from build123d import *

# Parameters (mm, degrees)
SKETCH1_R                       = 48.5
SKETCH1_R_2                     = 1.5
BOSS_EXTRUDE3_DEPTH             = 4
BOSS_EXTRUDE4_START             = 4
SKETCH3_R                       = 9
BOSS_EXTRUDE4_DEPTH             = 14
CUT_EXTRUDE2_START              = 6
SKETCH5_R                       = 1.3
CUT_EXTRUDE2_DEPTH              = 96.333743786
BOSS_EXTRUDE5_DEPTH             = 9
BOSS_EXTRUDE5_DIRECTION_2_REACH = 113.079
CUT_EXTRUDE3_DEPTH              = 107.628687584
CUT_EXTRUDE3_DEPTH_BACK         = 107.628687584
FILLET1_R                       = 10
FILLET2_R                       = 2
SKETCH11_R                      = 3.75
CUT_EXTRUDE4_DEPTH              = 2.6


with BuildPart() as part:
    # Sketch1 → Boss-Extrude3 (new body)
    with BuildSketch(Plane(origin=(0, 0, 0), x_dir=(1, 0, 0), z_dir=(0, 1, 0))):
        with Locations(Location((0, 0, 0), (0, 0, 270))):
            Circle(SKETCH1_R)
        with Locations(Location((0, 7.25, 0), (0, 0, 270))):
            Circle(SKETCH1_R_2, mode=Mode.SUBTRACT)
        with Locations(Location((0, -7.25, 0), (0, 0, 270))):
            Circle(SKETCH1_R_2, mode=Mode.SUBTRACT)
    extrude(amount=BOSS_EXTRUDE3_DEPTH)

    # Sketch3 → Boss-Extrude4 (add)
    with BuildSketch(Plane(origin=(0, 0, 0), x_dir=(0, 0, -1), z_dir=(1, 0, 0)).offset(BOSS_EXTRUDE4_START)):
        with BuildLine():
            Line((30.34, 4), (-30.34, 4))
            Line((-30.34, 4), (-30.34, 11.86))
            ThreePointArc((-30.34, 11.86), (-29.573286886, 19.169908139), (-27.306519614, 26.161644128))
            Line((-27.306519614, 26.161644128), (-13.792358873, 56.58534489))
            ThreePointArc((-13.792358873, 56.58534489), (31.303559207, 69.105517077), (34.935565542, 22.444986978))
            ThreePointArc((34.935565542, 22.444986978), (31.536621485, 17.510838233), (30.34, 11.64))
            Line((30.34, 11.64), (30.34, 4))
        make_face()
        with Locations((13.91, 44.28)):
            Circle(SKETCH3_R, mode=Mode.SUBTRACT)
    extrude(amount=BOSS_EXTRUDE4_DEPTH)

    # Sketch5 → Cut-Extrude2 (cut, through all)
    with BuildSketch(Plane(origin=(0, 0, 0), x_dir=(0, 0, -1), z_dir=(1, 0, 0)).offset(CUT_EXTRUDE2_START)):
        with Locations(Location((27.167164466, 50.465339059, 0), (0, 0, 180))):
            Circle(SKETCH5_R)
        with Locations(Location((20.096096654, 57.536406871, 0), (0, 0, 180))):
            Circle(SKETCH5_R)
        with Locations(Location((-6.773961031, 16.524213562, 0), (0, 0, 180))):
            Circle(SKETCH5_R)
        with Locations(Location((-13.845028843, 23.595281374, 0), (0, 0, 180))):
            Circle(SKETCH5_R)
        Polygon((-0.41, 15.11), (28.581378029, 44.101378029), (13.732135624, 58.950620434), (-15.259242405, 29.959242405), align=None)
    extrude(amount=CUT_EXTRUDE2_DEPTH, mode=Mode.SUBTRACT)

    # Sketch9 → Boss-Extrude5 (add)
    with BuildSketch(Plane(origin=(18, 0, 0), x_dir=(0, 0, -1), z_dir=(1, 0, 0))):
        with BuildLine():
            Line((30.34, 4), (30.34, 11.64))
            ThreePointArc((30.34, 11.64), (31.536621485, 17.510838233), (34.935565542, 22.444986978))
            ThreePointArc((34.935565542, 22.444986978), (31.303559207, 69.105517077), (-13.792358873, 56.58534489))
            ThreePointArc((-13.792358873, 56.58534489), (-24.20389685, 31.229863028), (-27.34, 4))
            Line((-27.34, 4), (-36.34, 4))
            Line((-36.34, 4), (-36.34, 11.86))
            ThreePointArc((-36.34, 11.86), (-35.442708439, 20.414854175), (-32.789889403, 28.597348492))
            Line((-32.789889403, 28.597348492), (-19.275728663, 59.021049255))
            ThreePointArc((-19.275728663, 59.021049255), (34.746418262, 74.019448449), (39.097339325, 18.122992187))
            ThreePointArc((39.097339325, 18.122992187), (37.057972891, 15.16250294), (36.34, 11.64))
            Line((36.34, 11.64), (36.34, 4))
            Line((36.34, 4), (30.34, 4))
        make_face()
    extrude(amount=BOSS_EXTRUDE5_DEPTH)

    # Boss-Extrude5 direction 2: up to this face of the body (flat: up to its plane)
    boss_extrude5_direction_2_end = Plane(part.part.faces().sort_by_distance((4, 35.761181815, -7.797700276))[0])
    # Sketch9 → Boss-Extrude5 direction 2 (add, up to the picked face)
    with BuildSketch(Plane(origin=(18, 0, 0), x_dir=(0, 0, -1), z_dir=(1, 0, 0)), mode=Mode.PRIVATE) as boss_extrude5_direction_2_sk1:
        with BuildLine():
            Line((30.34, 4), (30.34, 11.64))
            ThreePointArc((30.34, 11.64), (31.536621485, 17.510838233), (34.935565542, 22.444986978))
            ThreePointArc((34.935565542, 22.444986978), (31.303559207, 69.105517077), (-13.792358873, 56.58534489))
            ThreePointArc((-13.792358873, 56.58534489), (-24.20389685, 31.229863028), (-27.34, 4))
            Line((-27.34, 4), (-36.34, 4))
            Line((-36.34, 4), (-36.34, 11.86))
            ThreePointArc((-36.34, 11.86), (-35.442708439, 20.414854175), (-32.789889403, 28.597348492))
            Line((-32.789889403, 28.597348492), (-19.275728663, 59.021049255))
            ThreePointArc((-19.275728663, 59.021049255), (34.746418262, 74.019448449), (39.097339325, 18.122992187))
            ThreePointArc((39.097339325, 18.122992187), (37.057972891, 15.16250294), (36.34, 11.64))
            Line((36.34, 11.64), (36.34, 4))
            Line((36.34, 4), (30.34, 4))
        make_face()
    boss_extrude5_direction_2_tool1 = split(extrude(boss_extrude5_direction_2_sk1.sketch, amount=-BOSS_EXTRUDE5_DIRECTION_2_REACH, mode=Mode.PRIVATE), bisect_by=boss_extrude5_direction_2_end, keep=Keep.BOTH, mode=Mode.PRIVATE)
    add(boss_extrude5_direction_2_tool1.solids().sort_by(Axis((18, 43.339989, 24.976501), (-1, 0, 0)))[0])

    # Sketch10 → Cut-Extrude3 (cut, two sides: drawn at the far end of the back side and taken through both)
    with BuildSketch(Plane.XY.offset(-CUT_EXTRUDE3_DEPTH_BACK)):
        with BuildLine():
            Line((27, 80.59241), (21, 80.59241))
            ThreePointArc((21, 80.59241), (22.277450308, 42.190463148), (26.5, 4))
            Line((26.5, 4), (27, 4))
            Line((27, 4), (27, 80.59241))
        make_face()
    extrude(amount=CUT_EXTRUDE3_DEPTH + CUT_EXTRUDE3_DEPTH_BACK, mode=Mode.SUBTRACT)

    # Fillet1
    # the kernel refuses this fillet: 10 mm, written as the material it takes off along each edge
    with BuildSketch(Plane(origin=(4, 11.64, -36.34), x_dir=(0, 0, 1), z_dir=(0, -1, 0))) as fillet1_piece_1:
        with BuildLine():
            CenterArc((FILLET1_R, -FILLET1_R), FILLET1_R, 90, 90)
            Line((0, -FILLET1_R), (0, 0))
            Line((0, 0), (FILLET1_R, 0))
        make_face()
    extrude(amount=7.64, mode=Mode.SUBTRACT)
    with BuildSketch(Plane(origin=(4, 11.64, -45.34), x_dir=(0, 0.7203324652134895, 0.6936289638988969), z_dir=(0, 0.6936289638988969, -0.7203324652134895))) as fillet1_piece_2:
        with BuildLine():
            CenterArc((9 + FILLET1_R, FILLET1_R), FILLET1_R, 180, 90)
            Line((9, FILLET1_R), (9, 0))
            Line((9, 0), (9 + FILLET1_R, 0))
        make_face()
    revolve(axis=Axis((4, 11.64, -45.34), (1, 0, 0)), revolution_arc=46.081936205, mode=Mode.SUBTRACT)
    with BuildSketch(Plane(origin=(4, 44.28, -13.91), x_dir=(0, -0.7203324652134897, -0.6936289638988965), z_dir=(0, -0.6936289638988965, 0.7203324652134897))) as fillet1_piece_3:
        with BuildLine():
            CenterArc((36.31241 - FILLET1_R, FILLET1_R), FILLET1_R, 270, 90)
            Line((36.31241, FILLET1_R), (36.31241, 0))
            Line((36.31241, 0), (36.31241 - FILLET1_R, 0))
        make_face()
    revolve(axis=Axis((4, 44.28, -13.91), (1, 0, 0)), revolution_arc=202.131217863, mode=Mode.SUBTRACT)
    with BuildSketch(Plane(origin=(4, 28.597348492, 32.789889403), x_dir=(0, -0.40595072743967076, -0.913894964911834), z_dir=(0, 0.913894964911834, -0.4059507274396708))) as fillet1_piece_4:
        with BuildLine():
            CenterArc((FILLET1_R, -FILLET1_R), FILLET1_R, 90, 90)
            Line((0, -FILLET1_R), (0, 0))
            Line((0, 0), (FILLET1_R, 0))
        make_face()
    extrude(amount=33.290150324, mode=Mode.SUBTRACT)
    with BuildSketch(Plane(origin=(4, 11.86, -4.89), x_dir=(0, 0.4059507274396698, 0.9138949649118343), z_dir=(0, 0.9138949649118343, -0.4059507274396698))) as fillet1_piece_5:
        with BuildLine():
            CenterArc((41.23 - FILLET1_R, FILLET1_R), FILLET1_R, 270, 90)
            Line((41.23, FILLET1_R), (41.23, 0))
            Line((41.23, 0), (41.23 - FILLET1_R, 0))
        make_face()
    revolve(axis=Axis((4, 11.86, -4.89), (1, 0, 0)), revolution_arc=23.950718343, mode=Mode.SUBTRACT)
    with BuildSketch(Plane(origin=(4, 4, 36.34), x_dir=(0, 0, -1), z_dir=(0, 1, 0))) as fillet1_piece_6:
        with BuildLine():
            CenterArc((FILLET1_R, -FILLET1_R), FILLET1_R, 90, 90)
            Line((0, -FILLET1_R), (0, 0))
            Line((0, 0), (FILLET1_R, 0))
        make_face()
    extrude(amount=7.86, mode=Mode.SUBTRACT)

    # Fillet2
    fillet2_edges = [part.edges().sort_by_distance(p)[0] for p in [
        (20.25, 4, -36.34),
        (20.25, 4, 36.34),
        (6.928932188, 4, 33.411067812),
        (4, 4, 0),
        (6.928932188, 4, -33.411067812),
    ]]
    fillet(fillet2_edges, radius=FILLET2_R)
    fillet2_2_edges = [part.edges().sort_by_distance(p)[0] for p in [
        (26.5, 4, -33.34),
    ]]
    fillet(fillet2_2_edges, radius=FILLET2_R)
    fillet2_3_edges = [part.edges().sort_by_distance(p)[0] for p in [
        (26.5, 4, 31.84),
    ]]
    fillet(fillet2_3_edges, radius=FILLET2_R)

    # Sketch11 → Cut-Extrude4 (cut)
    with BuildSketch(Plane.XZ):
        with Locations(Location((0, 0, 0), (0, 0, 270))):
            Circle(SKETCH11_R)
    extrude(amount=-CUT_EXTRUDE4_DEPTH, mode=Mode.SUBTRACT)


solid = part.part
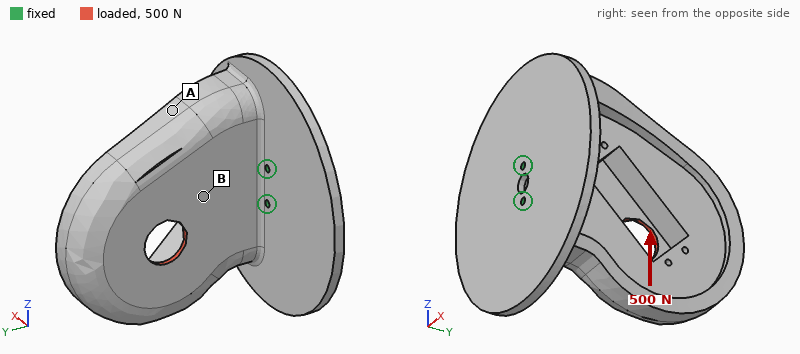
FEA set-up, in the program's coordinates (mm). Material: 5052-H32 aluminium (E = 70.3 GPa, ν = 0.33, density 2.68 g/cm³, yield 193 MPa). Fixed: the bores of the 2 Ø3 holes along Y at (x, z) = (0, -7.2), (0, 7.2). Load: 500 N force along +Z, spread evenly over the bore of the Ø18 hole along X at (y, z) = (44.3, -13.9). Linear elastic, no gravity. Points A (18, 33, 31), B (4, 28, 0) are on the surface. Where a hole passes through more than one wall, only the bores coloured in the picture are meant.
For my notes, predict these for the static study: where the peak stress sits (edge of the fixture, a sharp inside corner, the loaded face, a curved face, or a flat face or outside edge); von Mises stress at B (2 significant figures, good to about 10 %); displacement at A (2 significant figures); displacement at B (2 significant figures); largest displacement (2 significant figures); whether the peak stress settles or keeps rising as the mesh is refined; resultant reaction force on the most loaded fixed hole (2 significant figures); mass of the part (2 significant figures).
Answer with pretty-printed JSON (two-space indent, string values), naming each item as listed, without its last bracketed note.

{
  "where the peak stress sits": "edge of the fixture",
  "von Mises stress at B": "7.9 MPa",
  "displacement at A": "53 µm",
  "displacement at B": "34 µm",
  "largest displacement": "100 µm",
  "whether the peak stress settles or keeps rising as the mesh is refined": "keeps rising",
  "resultant reaction force on the most loaded fixed hole": "1.2 kN",
  "mass of the part": "250 g"
}
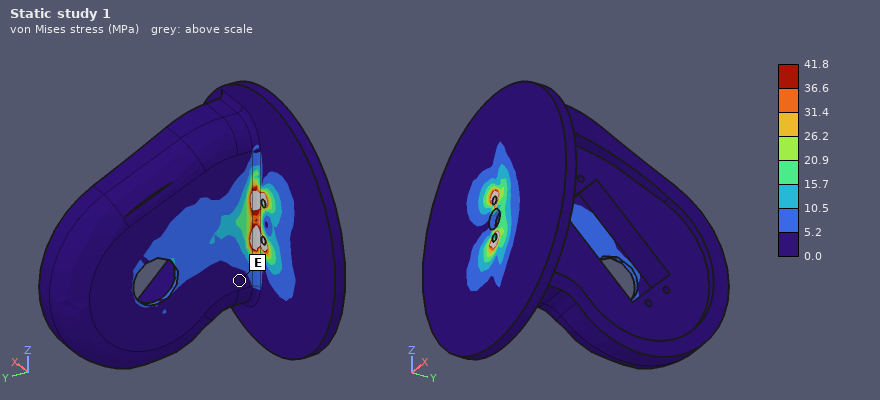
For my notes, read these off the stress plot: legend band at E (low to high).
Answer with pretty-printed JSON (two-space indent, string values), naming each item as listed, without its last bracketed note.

{
  "legend band at E": "0.0 to 5.2 MPa"
}
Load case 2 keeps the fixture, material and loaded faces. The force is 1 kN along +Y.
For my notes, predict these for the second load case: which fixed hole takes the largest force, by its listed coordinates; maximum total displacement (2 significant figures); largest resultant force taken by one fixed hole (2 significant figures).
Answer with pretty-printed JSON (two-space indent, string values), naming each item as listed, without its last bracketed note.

{
  "which fixed hole takes the largest force, by its listed coordinates": "(0, -7.2)",
  "maximum total displacement": "0.11 mm",
  "largest resultant force taken by one fixed hole": "1.2 kN"
}
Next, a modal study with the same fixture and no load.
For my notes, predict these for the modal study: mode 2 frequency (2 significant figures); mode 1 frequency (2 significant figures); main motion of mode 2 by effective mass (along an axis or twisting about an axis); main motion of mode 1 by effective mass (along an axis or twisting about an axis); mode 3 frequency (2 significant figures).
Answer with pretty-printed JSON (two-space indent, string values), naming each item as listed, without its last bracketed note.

{
  "mode 2 frequency": "1000 Hz",
  "mode 1 frequency": "440 Hz",
  "main motion of mode 2 by effective mass": "along Z",
  "main motion of mode 1 by effective mass": "along X",
  "mode 3 frequency": "1700 Hz"
}
